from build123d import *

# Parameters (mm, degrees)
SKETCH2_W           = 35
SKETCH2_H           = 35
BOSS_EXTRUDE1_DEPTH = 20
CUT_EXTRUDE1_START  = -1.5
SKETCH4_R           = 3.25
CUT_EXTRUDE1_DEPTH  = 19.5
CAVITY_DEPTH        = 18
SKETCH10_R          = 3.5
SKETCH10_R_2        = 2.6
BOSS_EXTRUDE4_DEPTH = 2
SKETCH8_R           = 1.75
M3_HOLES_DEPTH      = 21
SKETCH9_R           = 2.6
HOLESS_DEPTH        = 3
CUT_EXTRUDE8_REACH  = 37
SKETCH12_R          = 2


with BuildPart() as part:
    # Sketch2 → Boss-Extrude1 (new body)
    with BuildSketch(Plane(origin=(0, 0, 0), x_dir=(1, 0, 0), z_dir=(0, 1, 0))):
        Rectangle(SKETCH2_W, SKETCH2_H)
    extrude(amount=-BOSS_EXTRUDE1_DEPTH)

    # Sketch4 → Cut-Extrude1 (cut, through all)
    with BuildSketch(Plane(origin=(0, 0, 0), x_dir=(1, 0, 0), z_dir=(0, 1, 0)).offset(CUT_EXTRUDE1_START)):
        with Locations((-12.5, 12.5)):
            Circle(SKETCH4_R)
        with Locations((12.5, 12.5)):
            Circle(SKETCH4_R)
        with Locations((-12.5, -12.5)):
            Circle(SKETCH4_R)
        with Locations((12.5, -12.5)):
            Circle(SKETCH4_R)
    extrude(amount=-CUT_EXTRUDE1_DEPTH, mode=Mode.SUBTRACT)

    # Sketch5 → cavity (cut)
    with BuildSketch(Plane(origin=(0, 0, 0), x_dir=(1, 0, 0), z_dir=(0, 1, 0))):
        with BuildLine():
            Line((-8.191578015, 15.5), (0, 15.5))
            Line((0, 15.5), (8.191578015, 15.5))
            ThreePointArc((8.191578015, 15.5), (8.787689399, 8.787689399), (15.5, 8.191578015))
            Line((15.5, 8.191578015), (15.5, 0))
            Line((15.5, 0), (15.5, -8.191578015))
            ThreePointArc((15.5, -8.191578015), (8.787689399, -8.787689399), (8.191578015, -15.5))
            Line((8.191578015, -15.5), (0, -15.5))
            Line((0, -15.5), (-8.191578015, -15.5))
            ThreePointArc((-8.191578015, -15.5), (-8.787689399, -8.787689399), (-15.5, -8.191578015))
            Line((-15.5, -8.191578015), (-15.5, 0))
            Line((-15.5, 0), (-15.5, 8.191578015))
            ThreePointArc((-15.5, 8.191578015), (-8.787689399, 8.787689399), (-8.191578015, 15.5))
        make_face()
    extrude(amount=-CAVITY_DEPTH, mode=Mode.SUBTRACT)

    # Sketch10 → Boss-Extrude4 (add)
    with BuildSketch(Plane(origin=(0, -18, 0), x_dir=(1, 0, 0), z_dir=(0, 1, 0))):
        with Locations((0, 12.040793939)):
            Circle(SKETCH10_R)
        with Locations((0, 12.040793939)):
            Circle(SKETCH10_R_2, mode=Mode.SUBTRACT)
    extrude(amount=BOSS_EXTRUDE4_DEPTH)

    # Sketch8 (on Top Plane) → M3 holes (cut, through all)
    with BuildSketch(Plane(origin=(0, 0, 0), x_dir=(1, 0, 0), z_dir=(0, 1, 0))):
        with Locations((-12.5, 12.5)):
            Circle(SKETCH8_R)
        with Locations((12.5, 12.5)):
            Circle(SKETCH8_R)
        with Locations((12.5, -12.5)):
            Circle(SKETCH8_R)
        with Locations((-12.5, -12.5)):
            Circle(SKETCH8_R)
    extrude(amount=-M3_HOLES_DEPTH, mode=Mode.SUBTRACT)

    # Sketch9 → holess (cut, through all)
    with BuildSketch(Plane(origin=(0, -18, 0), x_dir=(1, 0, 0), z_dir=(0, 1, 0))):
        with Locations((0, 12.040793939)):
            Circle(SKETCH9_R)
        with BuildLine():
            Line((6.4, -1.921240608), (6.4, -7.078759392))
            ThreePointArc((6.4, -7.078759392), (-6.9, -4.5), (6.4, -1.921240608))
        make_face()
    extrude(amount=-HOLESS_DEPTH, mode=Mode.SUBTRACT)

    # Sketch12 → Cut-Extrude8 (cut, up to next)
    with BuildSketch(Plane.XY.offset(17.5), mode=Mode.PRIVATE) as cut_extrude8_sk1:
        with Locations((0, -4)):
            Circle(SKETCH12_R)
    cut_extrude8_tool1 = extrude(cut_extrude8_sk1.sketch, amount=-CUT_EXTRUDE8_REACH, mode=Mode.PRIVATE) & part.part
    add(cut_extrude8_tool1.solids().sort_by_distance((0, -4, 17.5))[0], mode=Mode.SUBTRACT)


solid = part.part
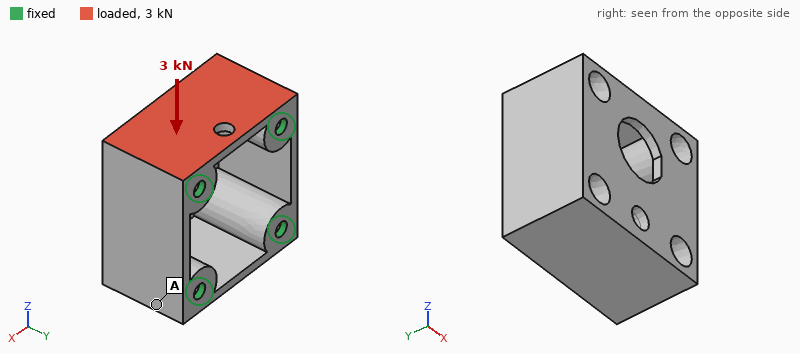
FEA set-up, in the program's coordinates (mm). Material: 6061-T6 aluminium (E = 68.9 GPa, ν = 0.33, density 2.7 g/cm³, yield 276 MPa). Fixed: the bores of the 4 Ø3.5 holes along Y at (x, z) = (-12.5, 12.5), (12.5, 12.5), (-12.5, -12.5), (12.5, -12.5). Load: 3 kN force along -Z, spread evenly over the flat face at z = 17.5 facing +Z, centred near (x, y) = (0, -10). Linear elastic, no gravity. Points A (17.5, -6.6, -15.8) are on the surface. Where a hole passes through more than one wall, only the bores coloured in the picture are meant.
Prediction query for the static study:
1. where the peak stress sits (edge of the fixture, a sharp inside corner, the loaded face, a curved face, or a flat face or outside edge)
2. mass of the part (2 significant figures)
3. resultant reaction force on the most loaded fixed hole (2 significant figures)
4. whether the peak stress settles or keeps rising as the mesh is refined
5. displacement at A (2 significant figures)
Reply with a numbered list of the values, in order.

1. edge of the fixture
2. 24 g
3. 1.2 kN
4. keeps rising
5. 12 µm
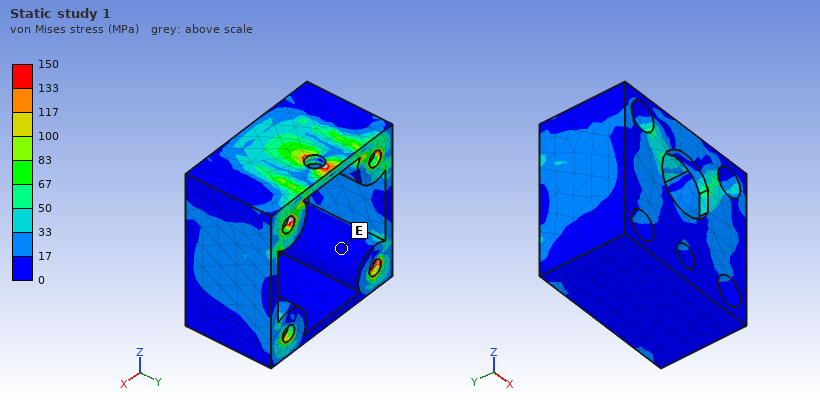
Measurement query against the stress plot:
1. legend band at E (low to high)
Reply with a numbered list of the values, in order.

1. 0 to 17 MPa
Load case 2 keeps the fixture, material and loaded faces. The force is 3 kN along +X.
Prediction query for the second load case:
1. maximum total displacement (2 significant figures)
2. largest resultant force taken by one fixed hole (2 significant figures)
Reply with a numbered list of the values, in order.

1. 44 µm
2. 1.5 kN
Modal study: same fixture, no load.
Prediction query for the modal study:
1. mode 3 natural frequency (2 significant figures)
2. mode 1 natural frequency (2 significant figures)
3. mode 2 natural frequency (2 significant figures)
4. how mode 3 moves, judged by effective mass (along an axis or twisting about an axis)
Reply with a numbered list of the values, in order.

1. 19 kHz
2. 12 kHz
3. 12 kHz
4. along Y
